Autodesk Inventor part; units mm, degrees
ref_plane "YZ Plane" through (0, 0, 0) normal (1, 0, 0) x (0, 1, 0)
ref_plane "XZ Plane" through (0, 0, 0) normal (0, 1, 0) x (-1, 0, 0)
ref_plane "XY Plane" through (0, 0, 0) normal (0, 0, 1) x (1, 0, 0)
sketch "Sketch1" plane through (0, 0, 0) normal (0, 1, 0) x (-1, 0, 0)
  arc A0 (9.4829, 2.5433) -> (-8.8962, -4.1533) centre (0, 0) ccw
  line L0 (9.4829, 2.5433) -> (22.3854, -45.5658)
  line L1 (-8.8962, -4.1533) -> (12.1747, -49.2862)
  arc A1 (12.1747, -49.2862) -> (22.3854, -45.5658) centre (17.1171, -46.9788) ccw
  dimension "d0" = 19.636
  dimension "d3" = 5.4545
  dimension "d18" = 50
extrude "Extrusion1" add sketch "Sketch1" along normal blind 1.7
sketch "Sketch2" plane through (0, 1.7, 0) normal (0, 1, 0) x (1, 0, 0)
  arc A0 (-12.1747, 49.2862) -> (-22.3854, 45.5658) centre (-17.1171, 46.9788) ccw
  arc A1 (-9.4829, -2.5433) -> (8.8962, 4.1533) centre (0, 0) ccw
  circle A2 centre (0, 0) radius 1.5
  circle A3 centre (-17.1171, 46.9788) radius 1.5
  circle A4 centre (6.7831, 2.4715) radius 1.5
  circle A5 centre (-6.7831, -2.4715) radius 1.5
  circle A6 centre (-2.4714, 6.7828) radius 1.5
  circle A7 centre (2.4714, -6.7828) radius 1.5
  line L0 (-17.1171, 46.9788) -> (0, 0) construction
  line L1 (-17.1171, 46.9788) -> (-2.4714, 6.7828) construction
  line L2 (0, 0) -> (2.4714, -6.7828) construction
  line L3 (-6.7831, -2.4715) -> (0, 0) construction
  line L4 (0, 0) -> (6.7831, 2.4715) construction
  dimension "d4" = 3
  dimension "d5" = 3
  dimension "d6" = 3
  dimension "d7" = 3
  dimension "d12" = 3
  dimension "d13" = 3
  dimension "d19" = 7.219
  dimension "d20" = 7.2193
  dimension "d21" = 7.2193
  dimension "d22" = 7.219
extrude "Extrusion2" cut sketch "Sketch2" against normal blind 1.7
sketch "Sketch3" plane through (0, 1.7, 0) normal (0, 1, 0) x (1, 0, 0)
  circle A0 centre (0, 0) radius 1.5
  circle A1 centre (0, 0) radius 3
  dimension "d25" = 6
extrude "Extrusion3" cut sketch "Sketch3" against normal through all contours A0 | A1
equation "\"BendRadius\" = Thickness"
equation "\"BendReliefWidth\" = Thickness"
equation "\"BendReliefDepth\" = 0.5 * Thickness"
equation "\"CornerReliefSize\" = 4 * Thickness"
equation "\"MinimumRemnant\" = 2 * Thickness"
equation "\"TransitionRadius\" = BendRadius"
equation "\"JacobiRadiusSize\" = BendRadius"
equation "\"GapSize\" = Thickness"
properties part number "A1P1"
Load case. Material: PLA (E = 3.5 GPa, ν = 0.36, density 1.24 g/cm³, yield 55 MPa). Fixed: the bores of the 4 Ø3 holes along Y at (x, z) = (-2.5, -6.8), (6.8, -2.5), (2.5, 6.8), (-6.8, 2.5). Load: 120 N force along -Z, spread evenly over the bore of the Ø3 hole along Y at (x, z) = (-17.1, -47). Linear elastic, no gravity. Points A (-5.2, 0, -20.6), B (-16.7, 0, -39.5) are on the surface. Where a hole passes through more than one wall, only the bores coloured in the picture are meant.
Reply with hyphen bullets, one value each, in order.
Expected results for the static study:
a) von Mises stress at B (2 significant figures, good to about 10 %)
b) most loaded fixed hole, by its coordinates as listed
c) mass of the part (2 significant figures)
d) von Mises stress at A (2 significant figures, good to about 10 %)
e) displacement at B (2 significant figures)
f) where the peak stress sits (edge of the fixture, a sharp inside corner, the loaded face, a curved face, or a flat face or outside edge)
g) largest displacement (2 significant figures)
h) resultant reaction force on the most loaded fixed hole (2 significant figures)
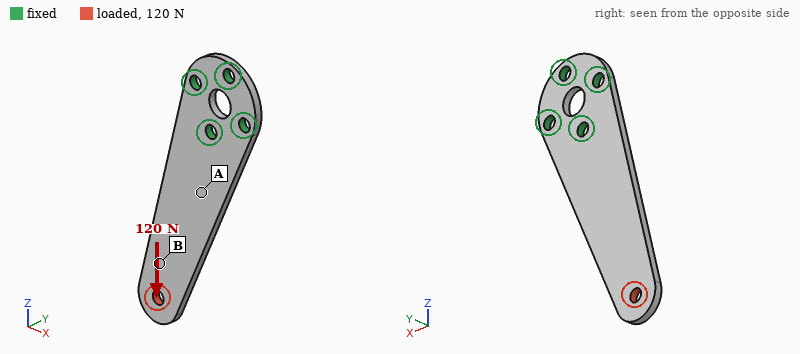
- 9.2 MPa
- (-6.8, 2.5)
- 1.9 g
- 2.6 MPa
- 0.52 mm
- edge of the fixture
- 0.82 mm
- 120 N
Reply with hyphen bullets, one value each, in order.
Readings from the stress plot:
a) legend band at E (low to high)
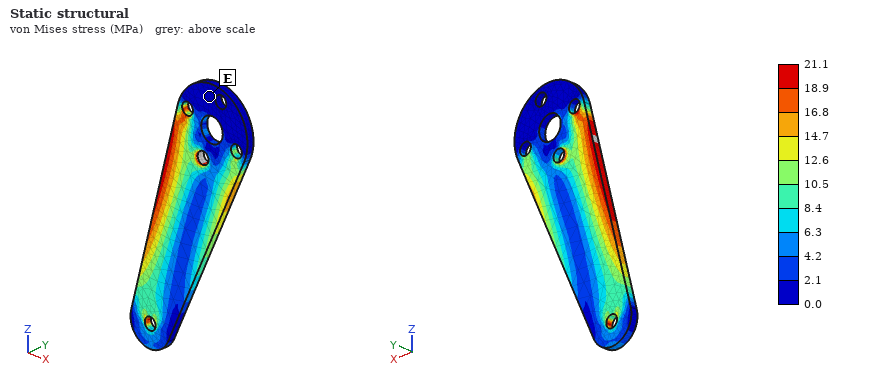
- 0.0 to 2.1 MPa
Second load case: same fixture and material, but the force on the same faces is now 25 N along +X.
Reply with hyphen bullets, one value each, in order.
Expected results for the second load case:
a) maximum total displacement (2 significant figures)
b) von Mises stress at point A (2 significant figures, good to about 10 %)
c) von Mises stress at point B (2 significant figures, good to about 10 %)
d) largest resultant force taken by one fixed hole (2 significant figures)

- 0.47 mm
- 3.2 MPa
- 2.5 MPa
- 58 N
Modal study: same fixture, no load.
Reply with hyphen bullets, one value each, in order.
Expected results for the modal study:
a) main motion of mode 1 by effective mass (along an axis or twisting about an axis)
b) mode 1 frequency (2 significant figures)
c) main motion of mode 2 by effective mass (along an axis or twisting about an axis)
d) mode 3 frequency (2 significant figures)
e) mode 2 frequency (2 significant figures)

- along Y
- 260 Hz
- along Y
- 1600 Hz
- 1400 Hz
